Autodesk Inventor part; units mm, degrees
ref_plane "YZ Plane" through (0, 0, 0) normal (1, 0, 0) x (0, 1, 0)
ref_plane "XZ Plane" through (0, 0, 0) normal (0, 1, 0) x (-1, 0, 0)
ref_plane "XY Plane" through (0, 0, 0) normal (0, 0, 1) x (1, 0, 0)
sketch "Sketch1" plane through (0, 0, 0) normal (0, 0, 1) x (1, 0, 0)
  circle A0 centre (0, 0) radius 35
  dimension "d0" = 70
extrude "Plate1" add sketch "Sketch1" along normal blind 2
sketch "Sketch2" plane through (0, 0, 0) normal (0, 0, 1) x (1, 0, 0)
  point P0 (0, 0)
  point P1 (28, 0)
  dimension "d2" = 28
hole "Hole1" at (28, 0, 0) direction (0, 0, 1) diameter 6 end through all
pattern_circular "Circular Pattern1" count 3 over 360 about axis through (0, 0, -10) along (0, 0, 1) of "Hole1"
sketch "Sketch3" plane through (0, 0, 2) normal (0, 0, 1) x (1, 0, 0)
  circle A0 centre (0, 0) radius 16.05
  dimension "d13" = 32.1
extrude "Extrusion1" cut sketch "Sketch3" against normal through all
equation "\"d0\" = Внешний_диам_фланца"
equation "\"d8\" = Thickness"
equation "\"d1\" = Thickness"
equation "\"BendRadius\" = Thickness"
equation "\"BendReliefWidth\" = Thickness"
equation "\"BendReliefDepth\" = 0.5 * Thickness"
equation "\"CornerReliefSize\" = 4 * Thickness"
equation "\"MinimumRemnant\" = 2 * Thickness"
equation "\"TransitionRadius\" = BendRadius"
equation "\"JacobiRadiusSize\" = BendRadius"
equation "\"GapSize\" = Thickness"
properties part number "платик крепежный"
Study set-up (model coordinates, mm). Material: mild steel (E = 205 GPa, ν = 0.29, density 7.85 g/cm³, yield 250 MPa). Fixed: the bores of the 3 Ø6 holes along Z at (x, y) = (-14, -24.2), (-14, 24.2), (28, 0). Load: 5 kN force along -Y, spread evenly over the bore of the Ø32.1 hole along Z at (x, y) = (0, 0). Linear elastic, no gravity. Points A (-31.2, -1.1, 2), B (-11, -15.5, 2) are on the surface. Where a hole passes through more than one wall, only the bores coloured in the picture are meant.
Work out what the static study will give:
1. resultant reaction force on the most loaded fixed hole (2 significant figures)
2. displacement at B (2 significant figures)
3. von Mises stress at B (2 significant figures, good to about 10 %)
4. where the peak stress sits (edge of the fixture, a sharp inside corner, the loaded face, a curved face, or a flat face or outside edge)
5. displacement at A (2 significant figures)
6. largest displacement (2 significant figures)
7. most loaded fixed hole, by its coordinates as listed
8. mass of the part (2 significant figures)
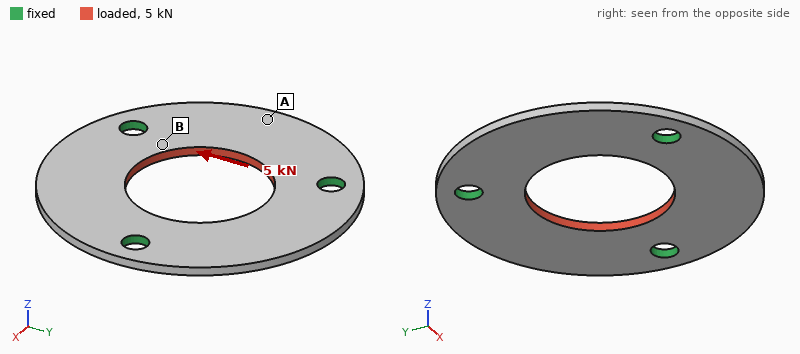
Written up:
2.0 kN
2.1 µm
49 MPa
edge of the fixture
1.6 µm
6.7 µm
(28, 0)
46 g
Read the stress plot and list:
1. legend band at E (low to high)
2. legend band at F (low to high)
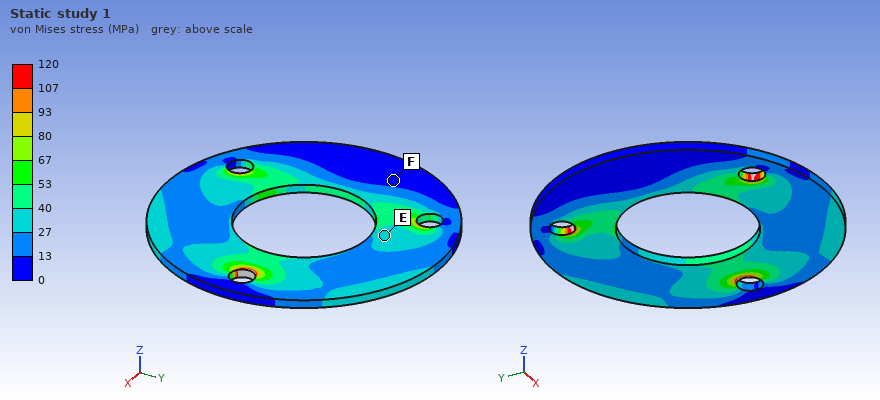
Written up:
27 to 40 MPa
0 to 13 MPa
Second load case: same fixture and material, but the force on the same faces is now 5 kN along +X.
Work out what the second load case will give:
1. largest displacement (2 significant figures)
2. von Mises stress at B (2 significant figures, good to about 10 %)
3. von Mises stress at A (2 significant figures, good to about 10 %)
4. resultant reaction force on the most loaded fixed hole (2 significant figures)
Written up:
7.5 µm
37 MPa
32 MPa
1.9 kN
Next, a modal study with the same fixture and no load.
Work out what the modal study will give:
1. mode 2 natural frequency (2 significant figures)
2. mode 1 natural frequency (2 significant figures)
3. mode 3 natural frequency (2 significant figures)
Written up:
3200 Hz
3200 Hz
3300 Hz
